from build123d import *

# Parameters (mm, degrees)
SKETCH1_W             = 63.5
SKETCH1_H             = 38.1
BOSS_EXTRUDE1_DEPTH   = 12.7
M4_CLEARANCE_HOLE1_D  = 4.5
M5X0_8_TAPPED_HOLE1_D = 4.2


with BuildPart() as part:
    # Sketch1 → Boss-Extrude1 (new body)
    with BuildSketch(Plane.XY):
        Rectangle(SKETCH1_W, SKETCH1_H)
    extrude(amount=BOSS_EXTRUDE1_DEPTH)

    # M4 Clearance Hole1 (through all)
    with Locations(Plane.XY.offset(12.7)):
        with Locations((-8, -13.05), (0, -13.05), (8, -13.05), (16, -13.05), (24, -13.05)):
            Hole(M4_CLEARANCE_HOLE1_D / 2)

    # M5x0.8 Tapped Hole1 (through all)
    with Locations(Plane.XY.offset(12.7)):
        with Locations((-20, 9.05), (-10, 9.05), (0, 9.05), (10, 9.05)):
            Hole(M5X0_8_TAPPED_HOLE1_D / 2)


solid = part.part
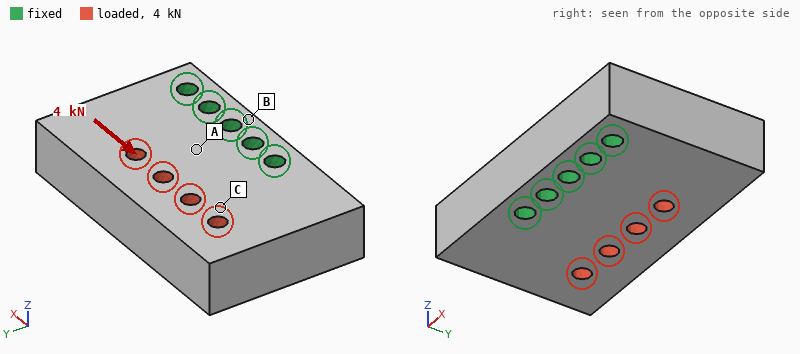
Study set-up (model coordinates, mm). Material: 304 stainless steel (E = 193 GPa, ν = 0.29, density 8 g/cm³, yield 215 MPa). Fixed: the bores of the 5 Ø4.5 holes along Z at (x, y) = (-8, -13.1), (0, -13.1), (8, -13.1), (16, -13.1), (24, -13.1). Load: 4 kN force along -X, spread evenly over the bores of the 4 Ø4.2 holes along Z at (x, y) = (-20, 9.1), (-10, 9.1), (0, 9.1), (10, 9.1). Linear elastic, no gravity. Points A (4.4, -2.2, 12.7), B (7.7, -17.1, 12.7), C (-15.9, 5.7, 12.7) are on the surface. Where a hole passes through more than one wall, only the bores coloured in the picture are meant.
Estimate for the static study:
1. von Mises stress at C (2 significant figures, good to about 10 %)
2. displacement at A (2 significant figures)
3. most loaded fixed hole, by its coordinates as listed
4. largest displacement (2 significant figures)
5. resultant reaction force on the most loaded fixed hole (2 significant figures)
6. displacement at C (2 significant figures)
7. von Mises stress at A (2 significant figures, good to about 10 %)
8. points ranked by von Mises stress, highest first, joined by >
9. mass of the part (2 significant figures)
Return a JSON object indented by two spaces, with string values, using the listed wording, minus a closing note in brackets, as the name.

{
  "von Mises stress at C": "8.3 MPa",
  "displacement at A": "1.3 µm",
  "most loaded fixed hole, by its coordinates as listed": "(-8, -13.1)",
  "largest displacement": "6.0 µm",
  "resultant reaction force on the most loaded fixed hole": "2.5 kN",
  "displacement at C": "3.5 µm",
  "von Mises stress at A": "17 MPa",
  "points ranked by von Mises stress, highest first, joined by >": "A > C > B",
  "mass of the part": "230 g"
}
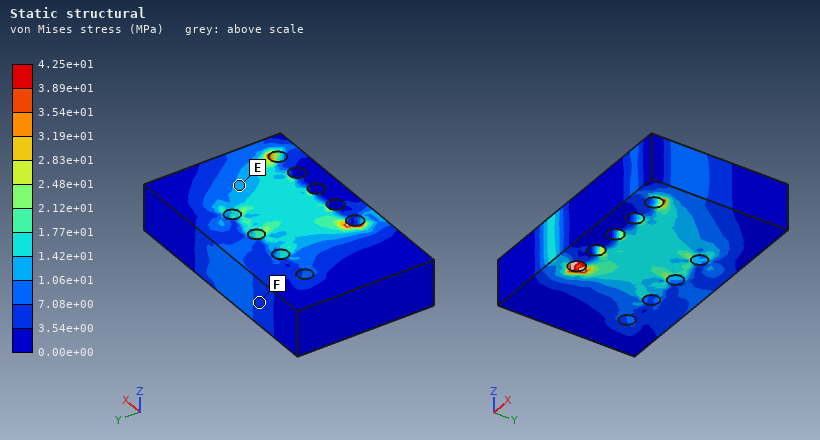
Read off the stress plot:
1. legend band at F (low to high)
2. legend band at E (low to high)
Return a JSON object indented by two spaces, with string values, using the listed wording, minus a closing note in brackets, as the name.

{
  "legend band at F": "3.54e+00 to 7.08e+00 MPa",
  "legend band at E": "1.06e+01 to 1.42e+01 MPa"
}
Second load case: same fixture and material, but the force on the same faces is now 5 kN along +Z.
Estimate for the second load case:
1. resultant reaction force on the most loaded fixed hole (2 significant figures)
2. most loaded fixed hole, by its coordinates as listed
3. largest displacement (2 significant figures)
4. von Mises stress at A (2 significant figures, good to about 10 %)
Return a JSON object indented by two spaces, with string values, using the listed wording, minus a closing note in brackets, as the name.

{
  "resultant reaction force on the most loaded fixed hole": "2.4 kN",
  "most loaded fixed hole, by its coordinates as listed": "(-8, -13.1)",
  "largest displacement": "30 µm",
  "von Mises stress at A": "44 MPa"
}
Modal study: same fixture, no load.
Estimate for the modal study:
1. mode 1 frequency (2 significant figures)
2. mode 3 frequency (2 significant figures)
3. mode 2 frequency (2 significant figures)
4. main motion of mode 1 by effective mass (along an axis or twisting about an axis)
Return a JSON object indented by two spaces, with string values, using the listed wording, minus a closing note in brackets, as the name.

{
  "mode 1 frequency": "7600 Hz",
  "mode 3 frequency": "12 kHz",
  "mode 2 frequency": "11 kHz",
  "main motion of mode 1 by effective mass": "along Z"
}
